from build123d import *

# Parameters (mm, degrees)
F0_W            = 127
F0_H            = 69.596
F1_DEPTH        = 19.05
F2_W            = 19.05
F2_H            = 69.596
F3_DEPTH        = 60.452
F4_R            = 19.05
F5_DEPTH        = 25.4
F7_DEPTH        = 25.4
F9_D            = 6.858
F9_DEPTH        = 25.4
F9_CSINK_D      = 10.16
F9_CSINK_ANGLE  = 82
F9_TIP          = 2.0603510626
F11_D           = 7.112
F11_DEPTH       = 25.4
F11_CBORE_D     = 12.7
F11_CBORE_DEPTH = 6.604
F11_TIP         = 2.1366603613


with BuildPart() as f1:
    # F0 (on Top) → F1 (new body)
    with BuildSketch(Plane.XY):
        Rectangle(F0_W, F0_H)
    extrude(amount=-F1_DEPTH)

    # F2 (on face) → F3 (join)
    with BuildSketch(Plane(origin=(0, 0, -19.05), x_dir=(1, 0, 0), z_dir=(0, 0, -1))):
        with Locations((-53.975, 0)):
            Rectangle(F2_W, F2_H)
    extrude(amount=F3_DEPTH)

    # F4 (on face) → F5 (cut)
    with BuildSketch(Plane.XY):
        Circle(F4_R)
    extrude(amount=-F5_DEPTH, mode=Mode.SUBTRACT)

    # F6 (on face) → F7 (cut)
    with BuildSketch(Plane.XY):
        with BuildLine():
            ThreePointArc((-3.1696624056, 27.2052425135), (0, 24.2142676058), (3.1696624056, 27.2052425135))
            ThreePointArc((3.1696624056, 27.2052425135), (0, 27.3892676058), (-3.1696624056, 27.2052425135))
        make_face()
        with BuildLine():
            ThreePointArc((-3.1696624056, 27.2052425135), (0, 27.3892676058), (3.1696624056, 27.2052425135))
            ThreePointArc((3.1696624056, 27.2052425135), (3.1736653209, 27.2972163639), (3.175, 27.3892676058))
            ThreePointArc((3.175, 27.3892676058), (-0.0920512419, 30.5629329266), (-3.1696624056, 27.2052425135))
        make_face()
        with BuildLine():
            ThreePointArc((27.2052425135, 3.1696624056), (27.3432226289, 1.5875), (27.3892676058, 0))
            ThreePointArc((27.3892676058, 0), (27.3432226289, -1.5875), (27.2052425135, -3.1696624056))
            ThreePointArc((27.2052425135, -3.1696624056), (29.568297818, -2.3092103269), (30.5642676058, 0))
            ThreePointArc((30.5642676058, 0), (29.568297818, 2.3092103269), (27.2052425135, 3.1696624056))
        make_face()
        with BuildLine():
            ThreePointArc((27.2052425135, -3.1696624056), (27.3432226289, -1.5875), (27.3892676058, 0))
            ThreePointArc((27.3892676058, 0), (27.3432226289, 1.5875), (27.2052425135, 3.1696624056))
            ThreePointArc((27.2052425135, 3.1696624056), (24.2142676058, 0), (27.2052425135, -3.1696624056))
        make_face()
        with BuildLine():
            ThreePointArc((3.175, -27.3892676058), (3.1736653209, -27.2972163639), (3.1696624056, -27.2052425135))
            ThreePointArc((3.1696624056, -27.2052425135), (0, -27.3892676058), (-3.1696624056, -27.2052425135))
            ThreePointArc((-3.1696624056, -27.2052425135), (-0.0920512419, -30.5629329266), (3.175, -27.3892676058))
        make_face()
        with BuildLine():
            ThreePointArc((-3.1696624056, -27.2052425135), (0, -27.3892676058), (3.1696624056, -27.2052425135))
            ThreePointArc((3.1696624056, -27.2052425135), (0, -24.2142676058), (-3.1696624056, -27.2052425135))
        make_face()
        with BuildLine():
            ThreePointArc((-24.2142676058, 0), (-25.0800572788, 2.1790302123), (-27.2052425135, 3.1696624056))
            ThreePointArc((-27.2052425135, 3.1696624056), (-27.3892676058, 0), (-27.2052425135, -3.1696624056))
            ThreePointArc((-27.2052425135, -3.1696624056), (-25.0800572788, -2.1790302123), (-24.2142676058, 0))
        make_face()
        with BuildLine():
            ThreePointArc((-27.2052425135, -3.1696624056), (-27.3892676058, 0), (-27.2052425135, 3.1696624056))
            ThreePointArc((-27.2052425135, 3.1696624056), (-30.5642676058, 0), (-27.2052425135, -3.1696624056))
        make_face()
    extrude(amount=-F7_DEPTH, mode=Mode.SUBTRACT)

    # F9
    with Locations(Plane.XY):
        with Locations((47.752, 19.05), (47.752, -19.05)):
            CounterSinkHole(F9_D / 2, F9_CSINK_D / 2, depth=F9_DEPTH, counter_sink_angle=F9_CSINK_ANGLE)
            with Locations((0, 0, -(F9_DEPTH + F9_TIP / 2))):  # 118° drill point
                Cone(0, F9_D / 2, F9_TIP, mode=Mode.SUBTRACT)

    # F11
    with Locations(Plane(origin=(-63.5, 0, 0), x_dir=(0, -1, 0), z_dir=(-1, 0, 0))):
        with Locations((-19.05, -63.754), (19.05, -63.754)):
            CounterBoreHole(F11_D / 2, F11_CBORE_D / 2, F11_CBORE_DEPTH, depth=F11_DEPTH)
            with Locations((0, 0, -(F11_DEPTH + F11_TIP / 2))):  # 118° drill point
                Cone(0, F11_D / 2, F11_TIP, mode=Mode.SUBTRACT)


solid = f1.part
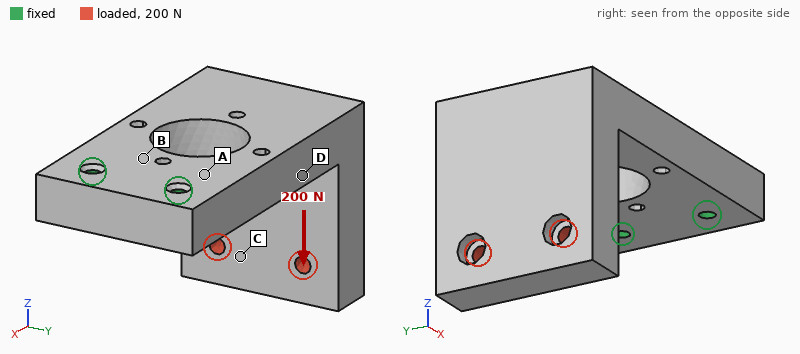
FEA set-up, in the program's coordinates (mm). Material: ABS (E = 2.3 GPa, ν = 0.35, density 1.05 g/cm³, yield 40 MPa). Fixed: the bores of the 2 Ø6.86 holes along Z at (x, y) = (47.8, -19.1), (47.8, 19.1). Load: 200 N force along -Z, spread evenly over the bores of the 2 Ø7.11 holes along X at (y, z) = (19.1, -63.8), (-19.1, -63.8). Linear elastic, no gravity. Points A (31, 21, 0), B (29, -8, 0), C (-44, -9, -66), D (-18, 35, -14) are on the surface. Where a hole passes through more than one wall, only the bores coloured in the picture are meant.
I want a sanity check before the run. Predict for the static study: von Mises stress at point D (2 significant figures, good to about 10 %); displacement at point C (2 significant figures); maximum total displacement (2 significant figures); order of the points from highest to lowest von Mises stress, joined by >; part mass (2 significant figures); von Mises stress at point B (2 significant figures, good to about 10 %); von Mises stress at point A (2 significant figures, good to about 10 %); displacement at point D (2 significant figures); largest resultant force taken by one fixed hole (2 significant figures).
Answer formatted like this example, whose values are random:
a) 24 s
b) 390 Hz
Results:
a) 1.7 MPa
b) 1.5 mm
c) 1.9 mm
d) A > B > D > C
e) 230 g
f) 2.9 MPa
g) 4.5 MPa
h) 0.57 mm
i) 100 N
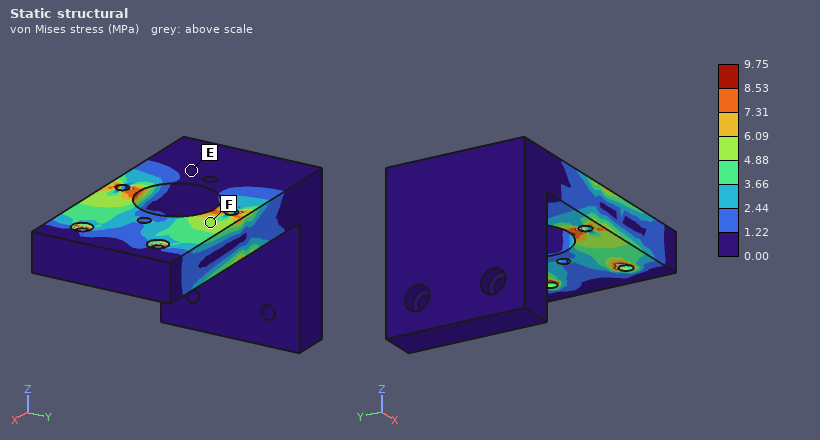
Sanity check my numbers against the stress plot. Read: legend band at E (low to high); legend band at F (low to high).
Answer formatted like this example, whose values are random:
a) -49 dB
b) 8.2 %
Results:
a) 0.00 to 1.22 MPa
b) 4.88 to 6.09 MPa
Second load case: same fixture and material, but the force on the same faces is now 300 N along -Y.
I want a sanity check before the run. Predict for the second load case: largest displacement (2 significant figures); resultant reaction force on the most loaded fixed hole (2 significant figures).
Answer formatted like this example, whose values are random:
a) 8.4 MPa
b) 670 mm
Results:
a) 1.6 mm
b) 770 N
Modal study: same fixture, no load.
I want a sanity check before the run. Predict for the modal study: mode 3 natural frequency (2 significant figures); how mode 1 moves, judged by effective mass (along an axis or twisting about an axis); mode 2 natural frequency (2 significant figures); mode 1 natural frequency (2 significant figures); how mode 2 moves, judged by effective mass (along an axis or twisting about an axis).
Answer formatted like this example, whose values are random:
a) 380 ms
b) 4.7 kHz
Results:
a) 610 Hz
b) along Z
c) 300 Hz
d) 160 Hz
e) along Y
